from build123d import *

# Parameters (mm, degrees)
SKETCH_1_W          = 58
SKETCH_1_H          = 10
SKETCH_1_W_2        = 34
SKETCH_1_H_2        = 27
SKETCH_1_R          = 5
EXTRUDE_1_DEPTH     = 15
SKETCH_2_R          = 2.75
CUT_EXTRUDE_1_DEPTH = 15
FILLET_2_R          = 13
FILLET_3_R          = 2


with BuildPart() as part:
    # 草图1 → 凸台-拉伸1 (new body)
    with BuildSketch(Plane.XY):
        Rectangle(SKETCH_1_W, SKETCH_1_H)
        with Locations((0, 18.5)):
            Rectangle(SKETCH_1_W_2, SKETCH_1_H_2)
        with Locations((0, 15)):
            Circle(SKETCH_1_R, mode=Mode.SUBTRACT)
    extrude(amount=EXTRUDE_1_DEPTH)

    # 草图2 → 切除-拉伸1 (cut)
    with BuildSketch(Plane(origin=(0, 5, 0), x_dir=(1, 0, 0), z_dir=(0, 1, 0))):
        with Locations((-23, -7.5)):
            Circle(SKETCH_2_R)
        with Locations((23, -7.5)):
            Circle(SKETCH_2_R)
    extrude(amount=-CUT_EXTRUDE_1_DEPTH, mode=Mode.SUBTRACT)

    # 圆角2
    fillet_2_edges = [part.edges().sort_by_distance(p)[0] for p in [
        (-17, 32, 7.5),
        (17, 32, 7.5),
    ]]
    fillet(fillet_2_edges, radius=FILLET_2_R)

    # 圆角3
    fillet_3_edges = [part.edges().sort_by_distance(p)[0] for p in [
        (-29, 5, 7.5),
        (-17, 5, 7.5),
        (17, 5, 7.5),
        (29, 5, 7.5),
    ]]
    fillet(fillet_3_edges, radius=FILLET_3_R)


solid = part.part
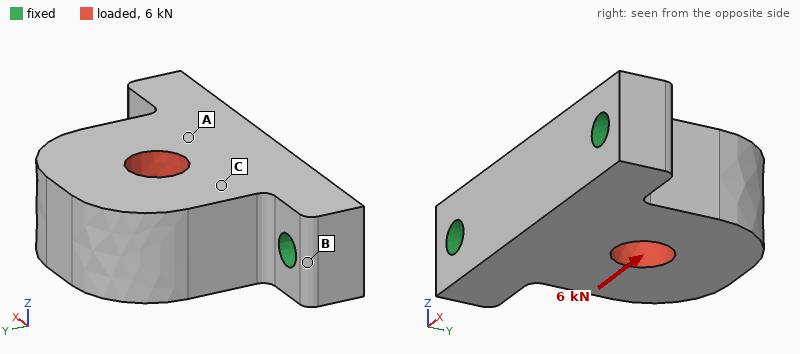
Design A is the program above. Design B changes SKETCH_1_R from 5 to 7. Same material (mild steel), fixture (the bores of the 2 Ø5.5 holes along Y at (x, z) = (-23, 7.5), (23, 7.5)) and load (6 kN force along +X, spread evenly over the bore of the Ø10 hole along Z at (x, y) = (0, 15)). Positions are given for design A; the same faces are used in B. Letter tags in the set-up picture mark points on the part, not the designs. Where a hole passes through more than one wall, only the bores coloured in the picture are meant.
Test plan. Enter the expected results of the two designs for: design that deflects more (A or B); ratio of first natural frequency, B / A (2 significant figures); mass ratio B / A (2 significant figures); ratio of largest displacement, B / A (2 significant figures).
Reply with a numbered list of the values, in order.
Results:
1. B
2. 1.0
3. 0.94
4. 1.2
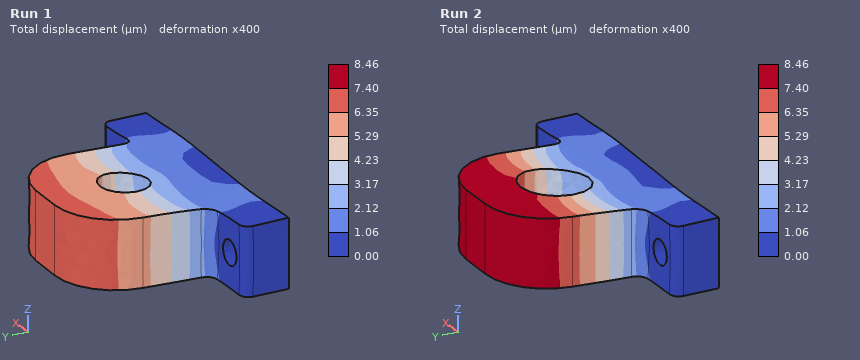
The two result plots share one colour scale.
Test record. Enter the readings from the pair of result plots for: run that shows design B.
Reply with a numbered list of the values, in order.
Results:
1. Run 2
